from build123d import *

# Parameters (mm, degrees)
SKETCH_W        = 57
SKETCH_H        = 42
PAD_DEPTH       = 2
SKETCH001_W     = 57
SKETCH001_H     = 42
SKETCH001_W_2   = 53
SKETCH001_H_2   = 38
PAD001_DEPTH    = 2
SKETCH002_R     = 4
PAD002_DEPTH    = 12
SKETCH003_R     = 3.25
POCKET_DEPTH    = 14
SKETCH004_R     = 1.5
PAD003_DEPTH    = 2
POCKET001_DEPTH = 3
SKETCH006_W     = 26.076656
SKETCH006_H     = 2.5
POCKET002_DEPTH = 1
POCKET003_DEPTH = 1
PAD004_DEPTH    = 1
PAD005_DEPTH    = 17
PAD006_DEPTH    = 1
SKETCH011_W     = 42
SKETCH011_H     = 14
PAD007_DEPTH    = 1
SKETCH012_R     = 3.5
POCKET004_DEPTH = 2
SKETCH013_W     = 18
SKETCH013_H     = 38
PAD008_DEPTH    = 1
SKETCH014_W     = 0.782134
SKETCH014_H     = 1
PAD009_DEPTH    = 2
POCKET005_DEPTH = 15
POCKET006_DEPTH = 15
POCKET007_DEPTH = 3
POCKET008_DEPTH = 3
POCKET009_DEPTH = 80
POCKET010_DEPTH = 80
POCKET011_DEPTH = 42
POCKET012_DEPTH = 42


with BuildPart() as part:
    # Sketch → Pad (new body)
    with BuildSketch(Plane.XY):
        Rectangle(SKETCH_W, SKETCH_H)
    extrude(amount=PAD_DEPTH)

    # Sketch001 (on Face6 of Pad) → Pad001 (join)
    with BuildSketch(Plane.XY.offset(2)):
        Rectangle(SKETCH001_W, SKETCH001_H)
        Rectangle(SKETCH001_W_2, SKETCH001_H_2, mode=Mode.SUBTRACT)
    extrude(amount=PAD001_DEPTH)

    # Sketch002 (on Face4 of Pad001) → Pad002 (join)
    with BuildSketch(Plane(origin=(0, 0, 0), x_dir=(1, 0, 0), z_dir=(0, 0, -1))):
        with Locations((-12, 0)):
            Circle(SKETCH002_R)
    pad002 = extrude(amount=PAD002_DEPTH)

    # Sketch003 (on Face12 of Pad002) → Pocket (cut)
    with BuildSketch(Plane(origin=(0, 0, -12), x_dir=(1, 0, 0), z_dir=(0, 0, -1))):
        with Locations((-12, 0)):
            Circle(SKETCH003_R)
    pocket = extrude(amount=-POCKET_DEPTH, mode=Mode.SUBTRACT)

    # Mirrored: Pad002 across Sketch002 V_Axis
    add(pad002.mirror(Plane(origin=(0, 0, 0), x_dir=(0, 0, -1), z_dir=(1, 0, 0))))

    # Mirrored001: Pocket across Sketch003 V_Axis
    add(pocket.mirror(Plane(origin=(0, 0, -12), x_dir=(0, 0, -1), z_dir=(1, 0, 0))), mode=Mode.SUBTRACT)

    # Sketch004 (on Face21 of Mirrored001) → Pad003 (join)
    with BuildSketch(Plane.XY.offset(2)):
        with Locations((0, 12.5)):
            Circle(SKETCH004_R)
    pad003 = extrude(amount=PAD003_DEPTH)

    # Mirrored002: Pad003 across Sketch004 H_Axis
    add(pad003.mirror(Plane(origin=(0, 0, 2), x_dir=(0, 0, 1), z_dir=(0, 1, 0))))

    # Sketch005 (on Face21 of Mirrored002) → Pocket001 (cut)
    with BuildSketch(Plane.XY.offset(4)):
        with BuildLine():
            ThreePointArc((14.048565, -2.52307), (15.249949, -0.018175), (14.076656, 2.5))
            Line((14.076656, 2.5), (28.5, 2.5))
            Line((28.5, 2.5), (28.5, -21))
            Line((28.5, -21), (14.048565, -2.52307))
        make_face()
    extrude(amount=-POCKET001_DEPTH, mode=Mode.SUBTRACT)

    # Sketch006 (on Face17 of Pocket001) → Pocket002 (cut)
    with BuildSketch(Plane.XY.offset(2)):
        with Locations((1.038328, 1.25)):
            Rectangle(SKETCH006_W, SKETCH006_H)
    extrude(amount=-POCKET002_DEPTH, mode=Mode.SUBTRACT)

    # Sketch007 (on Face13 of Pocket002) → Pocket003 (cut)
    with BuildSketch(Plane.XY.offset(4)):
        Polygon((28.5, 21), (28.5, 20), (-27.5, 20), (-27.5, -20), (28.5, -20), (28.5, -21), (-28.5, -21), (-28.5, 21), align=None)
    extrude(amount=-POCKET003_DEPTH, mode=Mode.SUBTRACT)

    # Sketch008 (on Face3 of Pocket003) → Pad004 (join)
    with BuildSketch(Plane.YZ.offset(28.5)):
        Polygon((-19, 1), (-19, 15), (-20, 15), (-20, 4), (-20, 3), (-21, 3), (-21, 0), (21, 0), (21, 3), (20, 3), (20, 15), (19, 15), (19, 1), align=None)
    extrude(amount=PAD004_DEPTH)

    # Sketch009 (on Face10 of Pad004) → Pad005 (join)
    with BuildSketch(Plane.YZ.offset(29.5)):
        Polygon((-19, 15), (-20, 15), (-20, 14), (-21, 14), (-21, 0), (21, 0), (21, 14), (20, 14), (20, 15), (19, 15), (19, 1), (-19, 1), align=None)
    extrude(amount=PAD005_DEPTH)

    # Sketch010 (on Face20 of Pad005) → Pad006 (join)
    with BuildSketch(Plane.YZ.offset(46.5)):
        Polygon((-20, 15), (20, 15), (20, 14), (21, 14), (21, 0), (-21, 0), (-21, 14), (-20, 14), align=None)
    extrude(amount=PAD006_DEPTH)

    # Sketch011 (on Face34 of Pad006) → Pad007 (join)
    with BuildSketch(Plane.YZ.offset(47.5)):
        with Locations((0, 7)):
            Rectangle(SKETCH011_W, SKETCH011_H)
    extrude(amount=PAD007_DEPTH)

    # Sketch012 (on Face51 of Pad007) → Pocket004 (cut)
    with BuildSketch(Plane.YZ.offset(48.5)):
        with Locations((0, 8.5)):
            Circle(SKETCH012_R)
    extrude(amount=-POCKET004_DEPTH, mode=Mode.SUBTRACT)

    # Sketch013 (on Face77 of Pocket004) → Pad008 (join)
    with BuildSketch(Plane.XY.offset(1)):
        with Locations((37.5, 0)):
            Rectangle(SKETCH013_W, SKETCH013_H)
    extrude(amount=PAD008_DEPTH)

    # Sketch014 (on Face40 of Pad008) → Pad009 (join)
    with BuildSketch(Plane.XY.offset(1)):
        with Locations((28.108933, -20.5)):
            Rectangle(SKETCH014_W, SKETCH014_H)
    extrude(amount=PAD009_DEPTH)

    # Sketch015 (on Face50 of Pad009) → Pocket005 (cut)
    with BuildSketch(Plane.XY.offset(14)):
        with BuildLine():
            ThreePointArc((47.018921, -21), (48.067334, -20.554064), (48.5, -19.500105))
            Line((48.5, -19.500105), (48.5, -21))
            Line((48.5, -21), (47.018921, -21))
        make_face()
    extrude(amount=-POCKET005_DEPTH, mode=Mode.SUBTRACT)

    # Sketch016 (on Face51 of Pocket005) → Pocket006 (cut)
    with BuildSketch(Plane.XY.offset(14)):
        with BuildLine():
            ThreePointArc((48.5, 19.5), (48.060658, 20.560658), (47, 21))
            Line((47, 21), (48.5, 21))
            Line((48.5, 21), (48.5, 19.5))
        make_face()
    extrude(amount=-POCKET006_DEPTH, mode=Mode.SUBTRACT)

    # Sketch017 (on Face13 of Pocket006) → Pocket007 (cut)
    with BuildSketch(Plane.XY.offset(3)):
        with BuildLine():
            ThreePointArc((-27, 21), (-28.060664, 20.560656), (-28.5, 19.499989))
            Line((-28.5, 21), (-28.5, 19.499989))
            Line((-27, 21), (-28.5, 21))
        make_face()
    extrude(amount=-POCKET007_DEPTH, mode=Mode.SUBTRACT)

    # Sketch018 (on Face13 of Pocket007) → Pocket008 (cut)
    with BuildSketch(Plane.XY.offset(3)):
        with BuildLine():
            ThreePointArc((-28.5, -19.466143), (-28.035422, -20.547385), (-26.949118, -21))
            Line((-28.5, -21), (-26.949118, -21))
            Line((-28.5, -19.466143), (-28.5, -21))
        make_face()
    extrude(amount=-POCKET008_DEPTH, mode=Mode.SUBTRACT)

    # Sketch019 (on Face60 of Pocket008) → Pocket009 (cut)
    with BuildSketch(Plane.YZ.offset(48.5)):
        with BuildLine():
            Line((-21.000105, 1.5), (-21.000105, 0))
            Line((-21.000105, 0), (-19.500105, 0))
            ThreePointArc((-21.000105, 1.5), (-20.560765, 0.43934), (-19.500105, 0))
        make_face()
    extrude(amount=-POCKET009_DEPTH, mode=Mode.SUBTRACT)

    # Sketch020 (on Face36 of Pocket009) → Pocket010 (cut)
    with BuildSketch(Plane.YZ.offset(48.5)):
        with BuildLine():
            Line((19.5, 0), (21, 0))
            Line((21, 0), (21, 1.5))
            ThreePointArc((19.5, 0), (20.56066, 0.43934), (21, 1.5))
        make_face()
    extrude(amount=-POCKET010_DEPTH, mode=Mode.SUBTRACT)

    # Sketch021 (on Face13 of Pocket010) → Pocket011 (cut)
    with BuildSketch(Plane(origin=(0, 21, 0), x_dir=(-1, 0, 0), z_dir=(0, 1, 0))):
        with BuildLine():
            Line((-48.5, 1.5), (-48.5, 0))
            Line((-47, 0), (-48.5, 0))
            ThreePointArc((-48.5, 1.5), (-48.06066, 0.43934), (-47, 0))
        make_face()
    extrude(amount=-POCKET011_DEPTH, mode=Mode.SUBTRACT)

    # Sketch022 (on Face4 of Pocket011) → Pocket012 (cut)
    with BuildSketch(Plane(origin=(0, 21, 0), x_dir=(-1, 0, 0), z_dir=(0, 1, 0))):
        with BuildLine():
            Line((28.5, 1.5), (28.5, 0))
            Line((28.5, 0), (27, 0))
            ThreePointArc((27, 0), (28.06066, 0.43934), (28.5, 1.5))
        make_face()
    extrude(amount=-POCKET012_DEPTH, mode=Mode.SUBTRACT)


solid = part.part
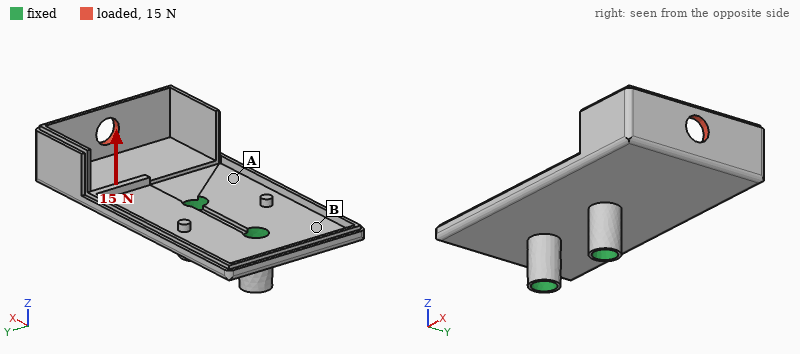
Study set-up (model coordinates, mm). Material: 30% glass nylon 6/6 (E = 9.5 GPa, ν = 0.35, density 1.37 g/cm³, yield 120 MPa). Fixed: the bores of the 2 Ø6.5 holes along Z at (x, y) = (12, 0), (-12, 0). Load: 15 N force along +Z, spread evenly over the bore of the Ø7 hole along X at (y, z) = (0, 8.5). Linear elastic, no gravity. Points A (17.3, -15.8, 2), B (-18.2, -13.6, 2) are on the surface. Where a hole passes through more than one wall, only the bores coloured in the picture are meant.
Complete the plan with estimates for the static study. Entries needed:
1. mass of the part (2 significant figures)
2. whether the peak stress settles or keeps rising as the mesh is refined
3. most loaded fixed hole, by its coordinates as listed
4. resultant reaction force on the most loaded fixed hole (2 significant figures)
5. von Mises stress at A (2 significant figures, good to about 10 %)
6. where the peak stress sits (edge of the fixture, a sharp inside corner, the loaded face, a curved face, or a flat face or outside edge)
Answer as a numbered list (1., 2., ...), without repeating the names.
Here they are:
1. 12 g
2. keeps rising
3. (12, 0)
4. 37 N
5. 7.4 MPa
6. a sharp inside corner
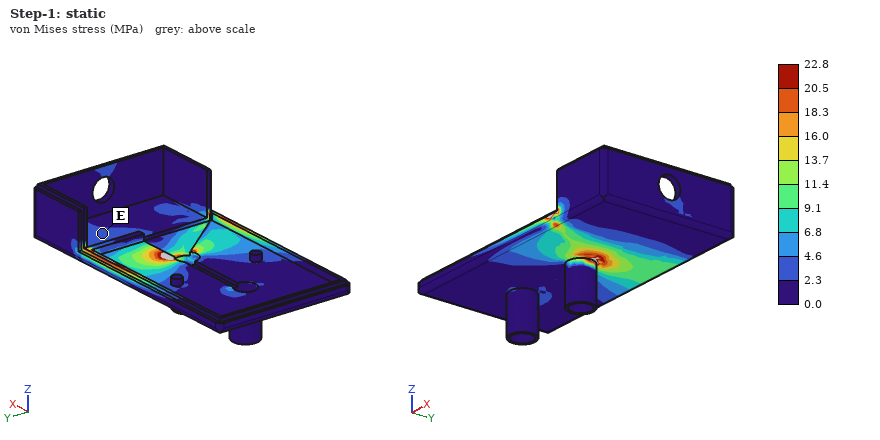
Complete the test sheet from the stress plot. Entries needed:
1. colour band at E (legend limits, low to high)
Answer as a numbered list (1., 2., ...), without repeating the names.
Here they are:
1. 2.3 to 4.6 MPa
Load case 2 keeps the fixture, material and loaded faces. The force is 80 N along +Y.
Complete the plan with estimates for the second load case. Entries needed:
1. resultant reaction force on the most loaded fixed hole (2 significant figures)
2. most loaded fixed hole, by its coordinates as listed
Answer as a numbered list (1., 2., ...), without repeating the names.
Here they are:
1. 170 N
2. (12, 0)
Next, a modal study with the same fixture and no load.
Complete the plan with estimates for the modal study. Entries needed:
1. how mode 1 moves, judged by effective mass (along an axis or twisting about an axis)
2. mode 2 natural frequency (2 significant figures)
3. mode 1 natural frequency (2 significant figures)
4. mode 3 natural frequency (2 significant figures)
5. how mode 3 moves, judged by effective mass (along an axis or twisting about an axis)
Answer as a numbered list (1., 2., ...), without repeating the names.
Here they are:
1. along Z
2. 640 Hz
3. 400 Hz
4. 1900 Hz
5. along Z
